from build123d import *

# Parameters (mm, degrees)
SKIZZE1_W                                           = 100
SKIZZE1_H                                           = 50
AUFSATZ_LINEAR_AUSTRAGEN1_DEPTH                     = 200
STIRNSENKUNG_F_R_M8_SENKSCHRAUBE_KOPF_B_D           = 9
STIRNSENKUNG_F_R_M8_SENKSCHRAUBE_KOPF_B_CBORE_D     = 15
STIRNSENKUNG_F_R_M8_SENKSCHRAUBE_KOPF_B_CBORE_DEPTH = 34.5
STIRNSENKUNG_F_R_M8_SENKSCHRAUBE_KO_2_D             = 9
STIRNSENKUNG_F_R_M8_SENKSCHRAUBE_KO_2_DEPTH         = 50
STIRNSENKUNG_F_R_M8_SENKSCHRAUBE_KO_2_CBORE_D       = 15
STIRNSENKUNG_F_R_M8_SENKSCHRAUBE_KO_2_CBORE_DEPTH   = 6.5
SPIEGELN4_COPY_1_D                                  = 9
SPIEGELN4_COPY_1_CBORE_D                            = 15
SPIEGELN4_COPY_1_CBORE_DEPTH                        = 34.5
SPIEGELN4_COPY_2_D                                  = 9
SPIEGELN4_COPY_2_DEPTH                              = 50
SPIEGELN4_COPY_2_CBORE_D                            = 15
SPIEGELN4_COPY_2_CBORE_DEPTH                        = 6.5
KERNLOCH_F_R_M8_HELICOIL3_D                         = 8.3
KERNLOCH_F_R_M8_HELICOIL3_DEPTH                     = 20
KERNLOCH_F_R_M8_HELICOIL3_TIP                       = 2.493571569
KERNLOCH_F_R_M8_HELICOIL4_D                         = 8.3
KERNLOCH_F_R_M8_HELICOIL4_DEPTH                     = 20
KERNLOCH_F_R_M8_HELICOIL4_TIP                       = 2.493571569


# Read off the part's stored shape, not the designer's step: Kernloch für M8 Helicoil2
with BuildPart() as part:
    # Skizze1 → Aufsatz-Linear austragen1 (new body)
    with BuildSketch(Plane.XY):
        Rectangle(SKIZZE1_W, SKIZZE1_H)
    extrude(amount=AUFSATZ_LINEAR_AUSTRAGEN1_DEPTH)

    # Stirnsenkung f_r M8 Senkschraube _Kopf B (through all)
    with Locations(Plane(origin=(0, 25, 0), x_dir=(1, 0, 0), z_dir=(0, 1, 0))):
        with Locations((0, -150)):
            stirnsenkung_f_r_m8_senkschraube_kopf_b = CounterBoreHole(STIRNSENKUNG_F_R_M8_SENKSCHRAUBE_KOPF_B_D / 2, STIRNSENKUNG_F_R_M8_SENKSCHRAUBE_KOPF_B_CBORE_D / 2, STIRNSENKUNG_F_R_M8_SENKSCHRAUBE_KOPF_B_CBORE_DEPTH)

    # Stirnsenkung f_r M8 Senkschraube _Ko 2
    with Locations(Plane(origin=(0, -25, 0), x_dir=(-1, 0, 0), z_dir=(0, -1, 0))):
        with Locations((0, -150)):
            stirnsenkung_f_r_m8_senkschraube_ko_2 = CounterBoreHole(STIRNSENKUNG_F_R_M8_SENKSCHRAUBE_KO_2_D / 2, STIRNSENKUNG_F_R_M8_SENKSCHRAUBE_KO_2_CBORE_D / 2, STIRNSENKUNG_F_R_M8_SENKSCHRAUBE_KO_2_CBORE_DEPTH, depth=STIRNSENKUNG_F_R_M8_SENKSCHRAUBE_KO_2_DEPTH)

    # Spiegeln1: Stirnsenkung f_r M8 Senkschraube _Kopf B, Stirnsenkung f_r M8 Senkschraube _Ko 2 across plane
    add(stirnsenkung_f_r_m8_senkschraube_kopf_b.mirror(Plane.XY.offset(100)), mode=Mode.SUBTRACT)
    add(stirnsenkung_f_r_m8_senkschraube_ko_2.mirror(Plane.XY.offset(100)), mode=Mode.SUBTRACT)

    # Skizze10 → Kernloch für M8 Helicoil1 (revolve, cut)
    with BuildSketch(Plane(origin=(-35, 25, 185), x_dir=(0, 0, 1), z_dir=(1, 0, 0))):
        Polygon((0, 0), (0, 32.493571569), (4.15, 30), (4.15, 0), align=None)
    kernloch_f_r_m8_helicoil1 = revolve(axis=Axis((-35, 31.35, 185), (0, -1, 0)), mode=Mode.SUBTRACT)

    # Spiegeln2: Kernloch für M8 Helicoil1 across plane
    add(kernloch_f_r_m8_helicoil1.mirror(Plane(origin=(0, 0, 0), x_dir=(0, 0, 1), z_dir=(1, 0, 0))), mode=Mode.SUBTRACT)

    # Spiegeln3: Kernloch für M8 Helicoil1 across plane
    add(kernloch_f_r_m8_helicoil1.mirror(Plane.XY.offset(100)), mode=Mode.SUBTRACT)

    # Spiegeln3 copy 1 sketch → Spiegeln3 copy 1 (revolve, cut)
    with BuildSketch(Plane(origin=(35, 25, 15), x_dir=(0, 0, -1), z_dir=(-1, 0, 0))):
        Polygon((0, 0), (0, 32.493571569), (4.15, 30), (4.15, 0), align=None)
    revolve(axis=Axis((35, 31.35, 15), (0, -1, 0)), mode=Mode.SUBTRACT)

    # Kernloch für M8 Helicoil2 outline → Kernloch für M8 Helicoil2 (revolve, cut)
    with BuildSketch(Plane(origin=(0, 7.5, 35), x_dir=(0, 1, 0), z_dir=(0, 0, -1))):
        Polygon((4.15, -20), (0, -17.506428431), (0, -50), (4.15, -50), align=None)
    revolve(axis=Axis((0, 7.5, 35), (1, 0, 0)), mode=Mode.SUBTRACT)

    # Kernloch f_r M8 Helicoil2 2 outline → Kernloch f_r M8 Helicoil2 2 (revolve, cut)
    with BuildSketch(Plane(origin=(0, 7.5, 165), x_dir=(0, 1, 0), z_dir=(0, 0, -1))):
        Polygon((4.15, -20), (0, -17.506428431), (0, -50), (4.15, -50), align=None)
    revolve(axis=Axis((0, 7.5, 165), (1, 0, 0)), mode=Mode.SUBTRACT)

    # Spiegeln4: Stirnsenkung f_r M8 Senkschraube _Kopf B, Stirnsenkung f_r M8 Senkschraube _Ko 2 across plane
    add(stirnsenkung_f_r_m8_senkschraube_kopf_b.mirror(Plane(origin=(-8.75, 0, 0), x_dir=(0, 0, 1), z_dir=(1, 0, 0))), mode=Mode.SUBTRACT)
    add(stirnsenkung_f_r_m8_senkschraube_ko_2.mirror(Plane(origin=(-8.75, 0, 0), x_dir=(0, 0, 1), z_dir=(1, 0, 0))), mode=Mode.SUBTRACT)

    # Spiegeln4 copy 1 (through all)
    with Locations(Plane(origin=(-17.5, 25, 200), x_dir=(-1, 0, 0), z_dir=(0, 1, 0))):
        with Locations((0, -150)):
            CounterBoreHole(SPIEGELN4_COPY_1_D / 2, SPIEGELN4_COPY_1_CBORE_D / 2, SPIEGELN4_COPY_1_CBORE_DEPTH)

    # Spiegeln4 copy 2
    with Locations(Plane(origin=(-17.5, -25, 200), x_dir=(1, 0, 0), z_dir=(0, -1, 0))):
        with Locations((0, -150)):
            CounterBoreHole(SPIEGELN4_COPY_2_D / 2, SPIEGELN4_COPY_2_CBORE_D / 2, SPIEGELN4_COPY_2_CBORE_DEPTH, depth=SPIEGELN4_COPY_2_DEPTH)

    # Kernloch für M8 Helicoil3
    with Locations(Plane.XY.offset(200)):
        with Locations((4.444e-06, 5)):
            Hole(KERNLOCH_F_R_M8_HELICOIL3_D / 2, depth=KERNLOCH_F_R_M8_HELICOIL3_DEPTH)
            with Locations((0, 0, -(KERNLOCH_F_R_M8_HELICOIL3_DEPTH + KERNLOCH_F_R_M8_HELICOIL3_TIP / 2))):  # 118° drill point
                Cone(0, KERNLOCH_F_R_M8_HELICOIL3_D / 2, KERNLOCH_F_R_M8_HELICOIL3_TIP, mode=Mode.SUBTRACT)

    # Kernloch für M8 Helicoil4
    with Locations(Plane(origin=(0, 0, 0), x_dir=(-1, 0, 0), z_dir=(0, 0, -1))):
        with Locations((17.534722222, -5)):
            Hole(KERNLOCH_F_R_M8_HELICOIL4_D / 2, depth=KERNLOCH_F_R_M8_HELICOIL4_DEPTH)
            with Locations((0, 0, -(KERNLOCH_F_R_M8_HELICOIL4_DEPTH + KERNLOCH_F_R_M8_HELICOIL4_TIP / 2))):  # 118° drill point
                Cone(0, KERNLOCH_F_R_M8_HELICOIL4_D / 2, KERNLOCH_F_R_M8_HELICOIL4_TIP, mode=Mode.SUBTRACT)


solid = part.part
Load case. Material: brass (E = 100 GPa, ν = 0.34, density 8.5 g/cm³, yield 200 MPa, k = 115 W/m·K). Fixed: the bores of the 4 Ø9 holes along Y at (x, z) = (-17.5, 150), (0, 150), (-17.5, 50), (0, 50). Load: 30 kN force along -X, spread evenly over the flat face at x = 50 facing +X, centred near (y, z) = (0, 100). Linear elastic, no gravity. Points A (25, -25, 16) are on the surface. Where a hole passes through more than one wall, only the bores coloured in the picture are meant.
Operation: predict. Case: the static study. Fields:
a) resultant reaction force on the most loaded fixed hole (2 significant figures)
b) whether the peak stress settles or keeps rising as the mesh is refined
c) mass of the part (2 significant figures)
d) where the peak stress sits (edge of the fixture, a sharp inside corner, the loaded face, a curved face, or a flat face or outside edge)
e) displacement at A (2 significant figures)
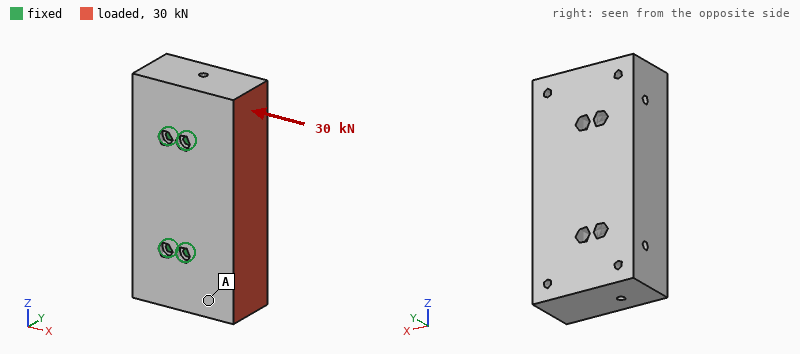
11 kN
keeps rising
8.1 kg
edge of the fixture
18 µm
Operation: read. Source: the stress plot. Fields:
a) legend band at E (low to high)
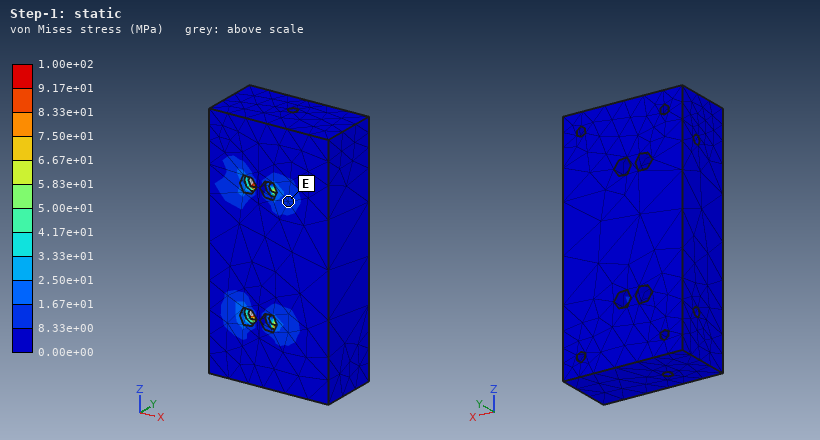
8.33e+00 to 1.67e+01 MPa
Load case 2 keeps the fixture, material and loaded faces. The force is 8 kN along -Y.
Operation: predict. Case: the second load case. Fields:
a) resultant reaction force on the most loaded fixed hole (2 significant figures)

11 kN
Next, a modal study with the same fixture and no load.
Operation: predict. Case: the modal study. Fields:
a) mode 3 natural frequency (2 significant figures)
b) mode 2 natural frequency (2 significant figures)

3100 Hz
2800 Hz
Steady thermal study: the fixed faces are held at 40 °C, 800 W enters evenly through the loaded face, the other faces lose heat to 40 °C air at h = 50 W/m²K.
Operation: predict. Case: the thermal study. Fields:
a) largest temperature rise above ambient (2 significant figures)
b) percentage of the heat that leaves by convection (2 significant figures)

71 K
18 %
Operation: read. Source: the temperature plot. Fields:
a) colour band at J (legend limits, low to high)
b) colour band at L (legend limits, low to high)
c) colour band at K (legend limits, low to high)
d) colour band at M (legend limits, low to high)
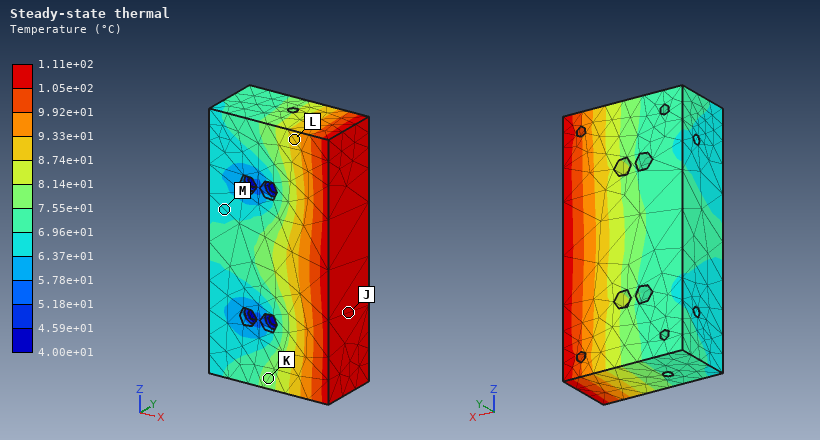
1.05e+02 to 1.11e+02 °C
8.74e+01 to 9.33e+01 °C
7.55e+01 to 8.14e+01 °C
6.37e+01 to 6.96e+01 °C
